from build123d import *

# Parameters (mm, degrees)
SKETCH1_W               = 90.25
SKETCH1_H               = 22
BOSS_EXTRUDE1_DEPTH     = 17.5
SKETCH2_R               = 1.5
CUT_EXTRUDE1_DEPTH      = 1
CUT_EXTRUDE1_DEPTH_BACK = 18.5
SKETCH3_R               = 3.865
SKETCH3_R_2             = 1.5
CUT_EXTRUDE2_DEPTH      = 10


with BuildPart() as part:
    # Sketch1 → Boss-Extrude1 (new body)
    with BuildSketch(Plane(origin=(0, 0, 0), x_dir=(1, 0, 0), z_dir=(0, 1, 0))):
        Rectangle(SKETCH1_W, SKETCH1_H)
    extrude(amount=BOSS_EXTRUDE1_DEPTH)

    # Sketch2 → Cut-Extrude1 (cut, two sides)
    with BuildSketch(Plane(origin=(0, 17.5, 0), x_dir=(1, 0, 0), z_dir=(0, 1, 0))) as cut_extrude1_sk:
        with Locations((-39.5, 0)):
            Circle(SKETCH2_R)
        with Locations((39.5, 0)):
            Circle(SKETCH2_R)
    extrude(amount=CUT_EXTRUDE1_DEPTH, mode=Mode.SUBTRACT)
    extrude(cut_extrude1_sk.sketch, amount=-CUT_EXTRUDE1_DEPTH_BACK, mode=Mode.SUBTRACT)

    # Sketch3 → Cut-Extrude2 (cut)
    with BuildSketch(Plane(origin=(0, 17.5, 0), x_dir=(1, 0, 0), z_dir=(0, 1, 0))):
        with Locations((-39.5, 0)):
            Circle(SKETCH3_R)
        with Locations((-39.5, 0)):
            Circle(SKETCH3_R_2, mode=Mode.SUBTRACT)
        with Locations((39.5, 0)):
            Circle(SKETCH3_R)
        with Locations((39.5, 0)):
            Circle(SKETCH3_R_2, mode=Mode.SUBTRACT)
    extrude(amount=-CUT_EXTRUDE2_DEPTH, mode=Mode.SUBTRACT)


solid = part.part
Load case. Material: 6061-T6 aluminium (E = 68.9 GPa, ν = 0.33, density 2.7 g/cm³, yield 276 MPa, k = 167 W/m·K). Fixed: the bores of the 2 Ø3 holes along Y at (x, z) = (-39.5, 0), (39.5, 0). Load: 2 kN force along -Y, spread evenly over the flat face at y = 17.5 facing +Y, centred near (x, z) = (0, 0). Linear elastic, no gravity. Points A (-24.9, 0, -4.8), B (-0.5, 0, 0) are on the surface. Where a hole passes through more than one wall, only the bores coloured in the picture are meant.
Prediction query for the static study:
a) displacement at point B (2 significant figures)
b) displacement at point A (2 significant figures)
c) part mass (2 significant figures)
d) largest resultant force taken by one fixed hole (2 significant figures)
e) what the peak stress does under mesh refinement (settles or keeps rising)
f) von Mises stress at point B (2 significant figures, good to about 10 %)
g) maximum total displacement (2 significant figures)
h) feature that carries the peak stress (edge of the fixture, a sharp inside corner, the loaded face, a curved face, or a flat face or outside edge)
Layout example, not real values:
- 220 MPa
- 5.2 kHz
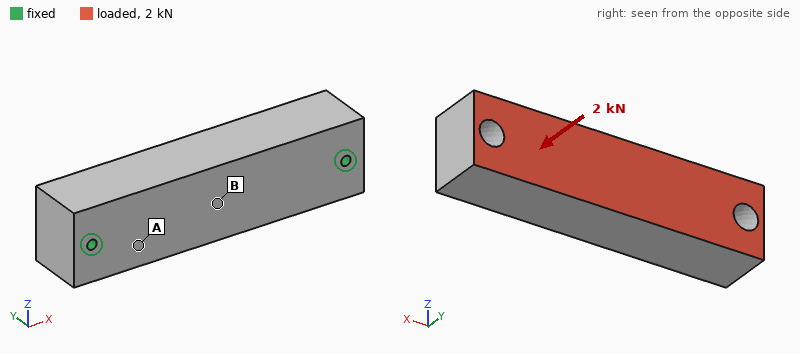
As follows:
- 12 µm
- 7.4 µm
- 91 g
- 1.2 kN
- keeps rising
- 7.9 MPa
- 13 µm
- edge of the fixture
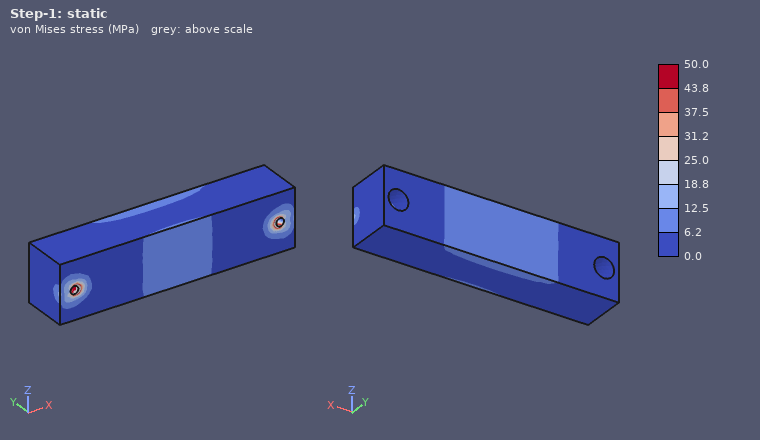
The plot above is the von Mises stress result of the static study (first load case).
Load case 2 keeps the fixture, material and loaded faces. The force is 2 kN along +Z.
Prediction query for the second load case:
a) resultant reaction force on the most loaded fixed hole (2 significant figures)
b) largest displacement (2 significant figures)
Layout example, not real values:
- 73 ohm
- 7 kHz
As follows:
- 1.0 kN
- 39 µm
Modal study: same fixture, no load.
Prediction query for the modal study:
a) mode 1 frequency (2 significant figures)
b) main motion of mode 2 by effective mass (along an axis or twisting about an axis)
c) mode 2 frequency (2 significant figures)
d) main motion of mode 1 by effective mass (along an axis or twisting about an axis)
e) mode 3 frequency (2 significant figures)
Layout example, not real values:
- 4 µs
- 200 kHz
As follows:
- 6300 Hz
- along Y
- 7400 Hz
- along Z
- 9600 Hz
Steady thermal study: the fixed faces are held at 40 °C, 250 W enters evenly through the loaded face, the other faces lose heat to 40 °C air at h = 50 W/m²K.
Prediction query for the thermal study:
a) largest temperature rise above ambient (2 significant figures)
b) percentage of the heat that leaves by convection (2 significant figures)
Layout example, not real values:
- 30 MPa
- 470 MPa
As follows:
- 63 K
- 5.1 %
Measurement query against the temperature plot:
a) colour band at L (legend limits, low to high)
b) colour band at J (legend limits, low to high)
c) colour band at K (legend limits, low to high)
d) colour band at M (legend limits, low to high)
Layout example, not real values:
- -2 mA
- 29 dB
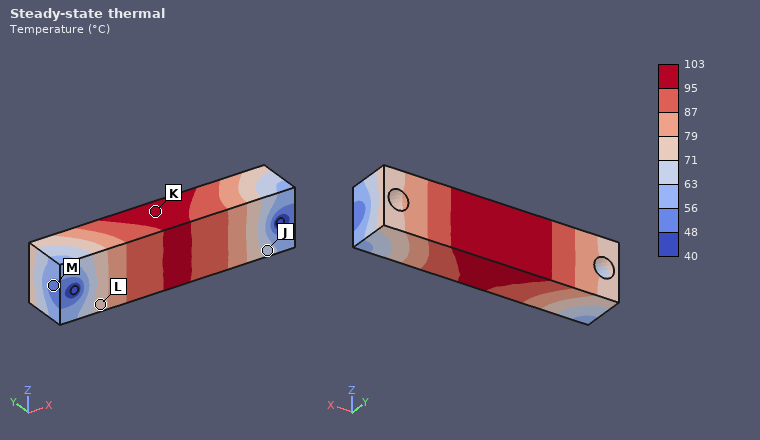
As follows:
- 71 to 79 °C
- 63 to 71 °C
- 95 to 103 °C
- 48 to 56 °C
